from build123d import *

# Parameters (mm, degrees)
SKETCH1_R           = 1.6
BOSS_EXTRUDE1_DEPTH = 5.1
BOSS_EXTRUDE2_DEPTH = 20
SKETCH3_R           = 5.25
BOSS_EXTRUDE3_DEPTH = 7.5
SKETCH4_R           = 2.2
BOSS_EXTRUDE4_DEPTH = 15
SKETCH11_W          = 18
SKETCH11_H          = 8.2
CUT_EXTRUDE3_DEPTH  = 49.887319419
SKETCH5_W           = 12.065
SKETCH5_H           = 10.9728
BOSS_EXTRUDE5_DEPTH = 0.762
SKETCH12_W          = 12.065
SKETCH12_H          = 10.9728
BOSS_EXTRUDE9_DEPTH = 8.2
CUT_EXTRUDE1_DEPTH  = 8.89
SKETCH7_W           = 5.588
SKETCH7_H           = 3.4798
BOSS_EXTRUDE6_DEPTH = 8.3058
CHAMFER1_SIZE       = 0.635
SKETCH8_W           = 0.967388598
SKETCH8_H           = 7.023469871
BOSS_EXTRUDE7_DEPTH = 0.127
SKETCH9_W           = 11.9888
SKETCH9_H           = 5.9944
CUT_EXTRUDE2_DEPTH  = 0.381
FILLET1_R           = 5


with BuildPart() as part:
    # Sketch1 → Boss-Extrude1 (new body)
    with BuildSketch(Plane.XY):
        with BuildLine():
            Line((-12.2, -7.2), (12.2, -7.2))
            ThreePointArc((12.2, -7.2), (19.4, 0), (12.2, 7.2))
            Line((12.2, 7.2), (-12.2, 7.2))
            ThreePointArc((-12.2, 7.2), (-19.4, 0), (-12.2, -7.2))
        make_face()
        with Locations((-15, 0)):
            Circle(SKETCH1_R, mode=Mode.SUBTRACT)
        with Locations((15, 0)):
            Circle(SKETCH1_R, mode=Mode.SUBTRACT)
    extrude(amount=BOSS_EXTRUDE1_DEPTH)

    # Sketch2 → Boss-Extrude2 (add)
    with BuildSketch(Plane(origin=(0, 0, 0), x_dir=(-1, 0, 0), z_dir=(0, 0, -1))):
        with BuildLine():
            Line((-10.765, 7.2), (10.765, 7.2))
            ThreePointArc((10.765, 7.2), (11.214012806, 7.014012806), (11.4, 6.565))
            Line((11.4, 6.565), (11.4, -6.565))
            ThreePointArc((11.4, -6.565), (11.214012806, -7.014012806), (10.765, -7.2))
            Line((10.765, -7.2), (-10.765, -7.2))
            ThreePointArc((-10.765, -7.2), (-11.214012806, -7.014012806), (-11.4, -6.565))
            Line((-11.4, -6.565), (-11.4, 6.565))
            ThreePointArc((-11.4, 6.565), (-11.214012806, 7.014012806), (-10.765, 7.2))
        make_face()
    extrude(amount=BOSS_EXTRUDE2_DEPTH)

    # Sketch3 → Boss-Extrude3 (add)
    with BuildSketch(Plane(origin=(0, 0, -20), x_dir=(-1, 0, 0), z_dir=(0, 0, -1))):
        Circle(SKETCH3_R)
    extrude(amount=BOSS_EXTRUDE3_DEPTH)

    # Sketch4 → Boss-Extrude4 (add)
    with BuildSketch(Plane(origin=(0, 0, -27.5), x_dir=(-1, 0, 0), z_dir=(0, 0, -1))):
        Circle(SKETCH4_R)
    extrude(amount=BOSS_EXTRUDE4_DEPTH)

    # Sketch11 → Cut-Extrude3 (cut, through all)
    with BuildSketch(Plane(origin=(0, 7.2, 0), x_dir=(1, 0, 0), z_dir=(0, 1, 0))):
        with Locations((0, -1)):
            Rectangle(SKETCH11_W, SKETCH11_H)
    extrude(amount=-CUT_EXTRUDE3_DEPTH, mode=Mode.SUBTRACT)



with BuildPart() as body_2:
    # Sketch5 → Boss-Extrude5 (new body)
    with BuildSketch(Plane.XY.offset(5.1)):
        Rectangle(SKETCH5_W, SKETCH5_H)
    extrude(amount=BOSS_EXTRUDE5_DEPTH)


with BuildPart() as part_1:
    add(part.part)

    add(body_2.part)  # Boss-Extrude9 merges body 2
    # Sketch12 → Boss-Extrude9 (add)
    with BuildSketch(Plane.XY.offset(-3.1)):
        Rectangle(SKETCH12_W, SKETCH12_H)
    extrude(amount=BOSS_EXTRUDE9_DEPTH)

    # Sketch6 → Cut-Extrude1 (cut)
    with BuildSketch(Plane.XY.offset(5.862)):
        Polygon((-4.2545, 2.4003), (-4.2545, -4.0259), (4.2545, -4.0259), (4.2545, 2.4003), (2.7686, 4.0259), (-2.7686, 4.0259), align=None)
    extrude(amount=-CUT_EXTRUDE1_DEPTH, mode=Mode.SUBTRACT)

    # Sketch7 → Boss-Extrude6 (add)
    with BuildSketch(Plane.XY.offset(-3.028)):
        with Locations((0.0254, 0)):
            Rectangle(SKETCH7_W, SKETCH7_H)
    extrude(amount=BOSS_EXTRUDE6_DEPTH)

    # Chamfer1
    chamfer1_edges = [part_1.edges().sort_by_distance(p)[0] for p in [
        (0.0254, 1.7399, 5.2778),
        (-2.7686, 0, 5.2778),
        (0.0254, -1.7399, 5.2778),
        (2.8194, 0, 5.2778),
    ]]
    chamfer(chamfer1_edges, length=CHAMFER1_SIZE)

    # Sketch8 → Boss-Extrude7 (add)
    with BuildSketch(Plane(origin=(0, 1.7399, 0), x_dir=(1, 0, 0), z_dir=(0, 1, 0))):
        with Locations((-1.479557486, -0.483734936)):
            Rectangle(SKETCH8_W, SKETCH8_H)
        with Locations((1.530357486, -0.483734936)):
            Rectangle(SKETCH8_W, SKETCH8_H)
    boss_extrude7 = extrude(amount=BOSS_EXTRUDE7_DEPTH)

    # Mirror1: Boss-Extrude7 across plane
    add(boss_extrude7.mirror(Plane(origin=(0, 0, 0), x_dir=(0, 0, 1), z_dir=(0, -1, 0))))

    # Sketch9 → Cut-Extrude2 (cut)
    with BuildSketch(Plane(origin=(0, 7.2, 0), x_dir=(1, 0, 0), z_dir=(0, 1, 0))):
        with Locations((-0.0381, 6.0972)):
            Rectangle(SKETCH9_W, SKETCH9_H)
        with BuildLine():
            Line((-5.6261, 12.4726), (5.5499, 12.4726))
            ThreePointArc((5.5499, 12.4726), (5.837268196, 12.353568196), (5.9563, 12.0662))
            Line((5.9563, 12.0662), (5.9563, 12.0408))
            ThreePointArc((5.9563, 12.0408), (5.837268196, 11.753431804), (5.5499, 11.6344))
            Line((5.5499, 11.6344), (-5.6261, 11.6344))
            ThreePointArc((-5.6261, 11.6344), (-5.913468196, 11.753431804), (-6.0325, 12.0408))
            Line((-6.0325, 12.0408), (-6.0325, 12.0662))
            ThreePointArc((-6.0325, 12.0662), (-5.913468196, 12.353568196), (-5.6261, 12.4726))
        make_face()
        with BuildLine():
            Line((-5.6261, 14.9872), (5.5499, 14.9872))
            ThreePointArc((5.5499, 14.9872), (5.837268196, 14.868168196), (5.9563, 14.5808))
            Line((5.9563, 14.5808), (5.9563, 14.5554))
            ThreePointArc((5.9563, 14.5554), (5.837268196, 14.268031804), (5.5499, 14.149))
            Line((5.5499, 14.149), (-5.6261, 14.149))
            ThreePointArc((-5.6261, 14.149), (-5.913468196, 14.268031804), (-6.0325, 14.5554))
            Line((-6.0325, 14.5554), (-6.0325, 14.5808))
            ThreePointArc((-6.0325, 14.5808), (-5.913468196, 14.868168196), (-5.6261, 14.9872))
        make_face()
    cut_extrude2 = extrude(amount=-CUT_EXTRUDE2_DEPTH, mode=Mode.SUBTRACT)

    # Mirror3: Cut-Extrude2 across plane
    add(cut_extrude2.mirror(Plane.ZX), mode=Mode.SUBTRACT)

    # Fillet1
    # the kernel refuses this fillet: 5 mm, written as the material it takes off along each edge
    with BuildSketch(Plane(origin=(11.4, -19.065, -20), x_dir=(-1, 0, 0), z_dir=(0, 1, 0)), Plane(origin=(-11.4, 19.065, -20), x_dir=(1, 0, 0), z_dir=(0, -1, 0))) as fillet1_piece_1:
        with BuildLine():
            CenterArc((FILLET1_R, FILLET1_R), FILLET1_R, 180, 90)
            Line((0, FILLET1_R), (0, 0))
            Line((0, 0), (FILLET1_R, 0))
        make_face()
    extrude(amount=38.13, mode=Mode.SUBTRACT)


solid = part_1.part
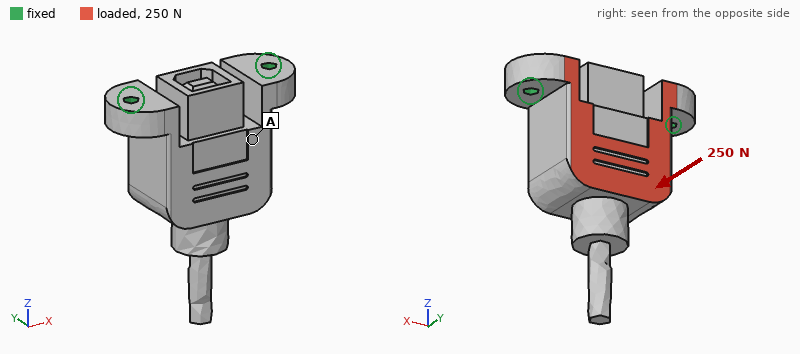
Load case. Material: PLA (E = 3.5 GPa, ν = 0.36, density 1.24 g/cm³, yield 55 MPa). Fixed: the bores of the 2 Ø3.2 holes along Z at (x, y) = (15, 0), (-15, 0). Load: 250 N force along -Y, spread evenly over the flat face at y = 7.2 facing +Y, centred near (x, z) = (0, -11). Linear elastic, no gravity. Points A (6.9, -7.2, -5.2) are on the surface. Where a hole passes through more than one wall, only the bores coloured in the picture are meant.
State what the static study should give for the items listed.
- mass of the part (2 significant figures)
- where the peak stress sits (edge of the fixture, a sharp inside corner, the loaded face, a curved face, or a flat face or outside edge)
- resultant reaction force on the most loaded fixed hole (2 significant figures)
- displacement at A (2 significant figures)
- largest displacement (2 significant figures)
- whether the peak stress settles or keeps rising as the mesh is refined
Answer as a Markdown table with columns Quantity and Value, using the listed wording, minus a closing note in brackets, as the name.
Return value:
| Quantity | Value |
|---|---|
| mass of the part | 10 g |
| where the peak stress sits | edge of the fixture |
| resultant reaction force on the most loaded fixed hole | 130 N |
| displacement at A | 0.18 mm |
| largest displacement | 0.74 mm |
| whether the peak stress settles or keeps rising as the mesh is refined | keeps rising |
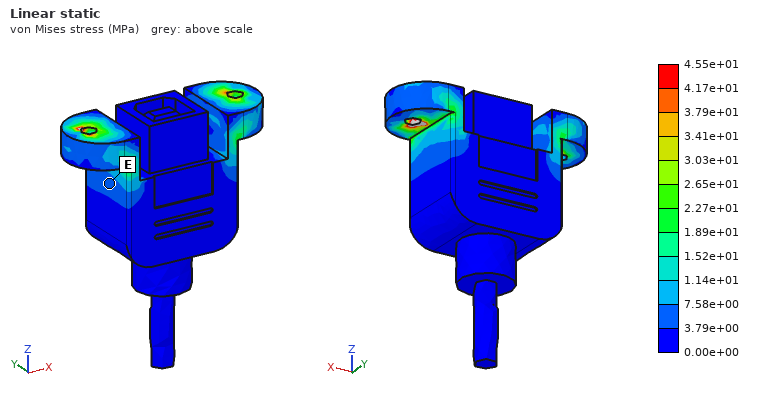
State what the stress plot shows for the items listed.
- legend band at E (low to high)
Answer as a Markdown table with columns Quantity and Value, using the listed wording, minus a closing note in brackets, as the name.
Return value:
| Quantity | Value |
|---|---|
| legend band at E | 3.79e+00 to 7.58e+00 MPa |
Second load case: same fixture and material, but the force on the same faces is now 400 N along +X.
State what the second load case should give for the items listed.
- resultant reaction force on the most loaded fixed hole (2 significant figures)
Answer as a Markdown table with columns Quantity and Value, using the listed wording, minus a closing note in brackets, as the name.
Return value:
| Quantity | Value |
|---|---|
| resultant reaction force on the most loaded fixed hole | 290 N |
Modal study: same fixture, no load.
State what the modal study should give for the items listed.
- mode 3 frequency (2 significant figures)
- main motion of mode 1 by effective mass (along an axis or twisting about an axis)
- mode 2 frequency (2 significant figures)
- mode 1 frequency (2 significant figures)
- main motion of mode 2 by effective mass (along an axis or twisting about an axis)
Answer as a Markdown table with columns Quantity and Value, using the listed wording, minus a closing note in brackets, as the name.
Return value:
| Quantity | Value |
|---|---|
| mode 3 frequency | 4000 Hz |
| main motion of mode 1 by effective mass | along Y |
| mode 2 frequency | 3300 Hz |
| mode 1 frequency | 1400 Hz |
| main motion of mode 2 by effective mass | along X |
